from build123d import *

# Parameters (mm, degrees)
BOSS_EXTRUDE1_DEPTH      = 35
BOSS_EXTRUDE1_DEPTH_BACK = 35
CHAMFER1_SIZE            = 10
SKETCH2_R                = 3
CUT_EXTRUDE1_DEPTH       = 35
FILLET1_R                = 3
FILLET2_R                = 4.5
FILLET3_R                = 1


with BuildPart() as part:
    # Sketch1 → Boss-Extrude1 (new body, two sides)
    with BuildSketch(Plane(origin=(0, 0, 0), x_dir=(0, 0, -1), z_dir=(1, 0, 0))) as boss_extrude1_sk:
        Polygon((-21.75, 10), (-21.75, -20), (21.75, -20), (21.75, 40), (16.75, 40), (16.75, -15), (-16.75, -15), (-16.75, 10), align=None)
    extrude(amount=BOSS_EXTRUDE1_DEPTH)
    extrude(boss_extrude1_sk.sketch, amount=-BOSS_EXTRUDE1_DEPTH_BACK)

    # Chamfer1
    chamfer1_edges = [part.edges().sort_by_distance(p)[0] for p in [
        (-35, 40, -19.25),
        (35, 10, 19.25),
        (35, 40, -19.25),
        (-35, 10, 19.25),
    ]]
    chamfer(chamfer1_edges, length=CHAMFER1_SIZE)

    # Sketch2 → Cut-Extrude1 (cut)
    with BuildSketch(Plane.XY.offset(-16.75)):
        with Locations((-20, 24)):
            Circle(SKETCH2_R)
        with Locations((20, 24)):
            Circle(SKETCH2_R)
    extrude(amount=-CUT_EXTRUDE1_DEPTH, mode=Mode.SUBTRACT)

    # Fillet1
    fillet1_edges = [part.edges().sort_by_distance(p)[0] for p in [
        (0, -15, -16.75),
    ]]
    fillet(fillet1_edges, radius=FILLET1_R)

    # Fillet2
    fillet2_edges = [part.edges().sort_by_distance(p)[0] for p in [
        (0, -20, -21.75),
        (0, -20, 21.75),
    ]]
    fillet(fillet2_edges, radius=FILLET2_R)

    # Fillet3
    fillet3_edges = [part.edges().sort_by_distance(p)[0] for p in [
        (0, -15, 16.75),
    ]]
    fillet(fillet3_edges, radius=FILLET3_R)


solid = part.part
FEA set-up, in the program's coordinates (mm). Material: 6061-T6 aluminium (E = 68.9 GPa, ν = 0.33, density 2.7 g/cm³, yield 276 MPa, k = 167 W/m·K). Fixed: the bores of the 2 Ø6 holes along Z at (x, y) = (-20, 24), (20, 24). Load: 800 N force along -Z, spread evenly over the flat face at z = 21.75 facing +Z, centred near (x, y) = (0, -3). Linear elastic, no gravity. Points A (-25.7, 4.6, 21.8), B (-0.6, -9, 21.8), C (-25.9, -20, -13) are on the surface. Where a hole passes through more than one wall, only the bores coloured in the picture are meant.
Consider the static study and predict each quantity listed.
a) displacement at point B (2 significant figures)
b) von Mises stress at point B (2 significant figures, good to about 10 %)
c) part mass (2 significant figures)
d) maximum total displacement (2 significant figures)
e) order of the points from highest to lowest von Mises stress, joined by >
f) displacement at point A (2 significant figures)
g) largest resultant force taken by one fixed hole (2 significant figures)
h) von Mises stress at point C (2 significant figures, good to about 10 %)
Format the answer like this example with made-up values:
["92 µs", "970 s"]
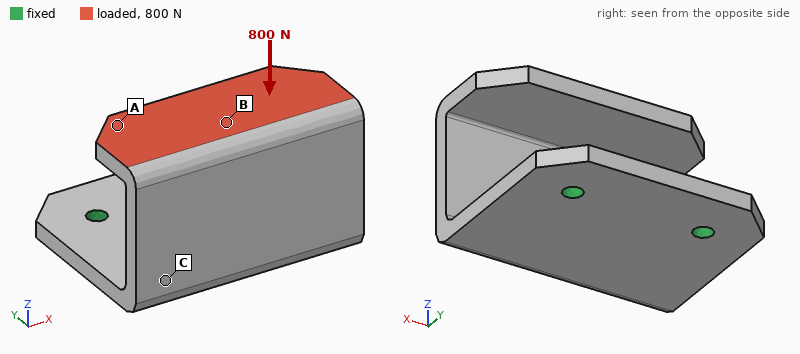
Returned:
["0.22 mm", "18 MPa", "110 g", "0.30 mm", "C > B > A", "0.27 mm", "400 N", "32 MPa"]
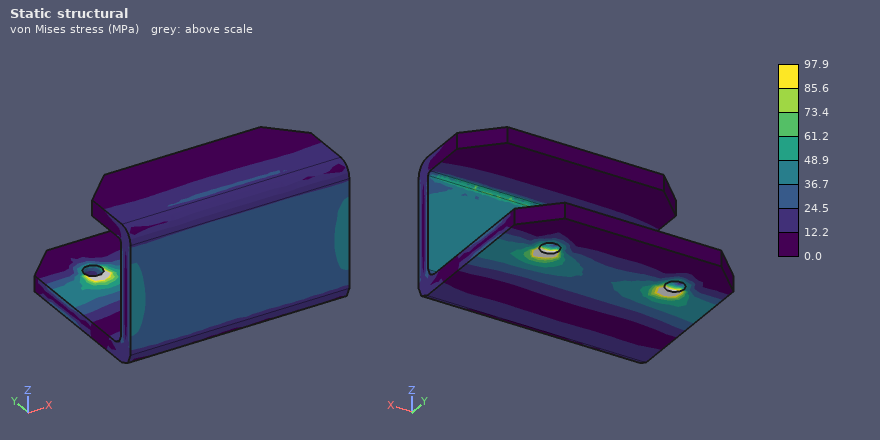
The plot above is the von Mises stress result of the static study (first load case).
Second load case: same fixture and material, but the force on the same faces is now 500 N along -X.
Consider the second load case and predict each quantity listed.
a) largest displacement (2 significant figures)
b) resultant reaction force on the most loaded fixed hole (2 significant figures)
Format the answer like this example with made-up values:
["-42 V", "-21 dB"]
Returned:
["0.39 mm", "580 N"]
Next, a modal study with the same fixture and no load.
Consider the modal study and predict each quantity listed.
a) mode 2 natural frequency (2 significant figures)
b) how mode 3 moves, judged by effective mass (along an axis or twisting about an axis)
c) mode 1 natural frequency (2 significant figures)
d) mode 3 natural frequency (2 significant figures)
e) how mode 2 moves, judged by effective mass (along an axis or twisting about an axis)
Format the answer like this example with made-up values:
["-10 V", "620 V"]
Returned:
["1000 Hz", "along Z", "620 Hz", "1400 Hz", "along X"]
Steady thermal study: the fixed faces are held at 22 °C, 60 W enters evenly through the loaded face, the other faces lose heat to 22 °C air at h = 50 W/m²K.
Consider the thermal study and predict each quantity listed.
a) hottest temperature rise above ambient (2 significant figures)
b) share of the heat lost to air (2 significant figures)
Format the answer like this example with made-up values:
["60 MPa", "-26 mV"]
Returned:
["68 K", "40 %"]
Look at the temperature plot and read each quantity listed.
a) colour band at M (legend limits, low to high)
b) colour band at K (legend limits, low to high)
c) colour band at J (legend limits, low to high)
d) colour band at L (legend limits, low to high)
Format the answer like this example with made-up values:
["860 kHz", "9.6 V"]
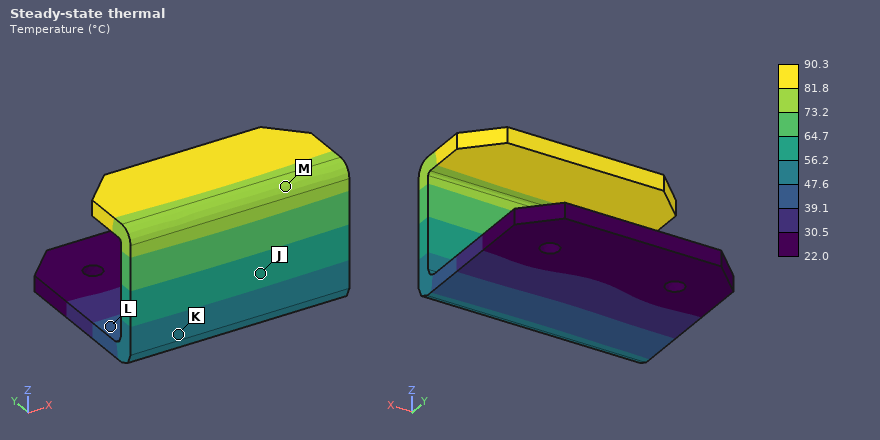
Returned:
["73.2 to 81.8 °C", "47.6 to 56.2 °C", "56.2 to 64.7 °C", "39.1 to 47.6 °C"]
